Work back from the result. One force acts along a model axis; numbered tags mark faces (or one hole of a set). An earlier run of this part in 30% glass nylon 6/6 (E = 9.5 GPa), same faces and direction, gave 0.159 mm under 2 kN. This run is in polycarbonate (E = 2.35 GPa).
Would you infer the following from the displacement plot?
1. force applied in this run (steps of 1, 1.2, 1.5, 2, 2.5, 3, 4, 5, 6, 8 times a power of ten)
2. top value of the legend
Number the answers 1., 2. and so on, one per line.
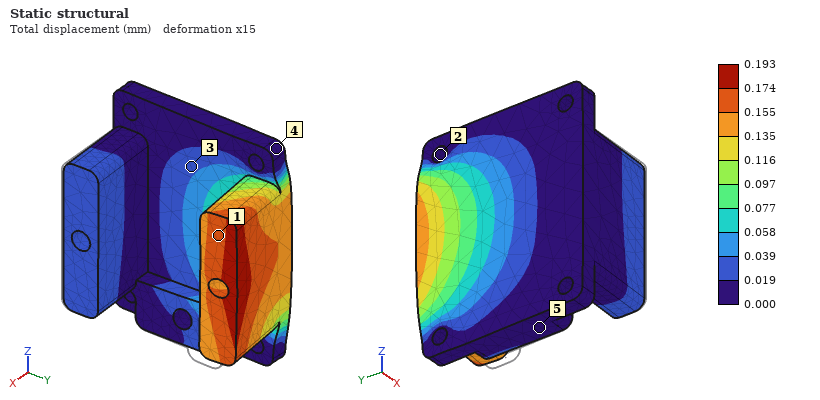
1. 600 N
2. 0.193 mm
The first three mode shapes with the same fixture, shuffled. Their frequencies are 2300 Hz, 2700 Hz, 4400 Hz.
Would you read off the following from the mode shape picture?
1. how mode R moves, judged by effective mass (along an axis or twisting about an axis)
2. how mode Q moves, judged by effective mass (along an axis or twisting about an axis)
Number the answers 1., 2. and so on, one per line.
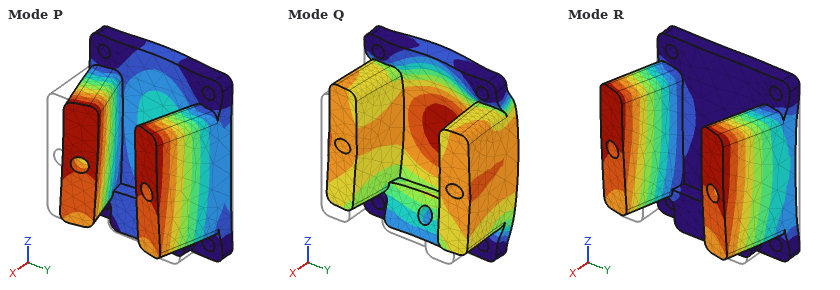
1. along Y
2. along X
